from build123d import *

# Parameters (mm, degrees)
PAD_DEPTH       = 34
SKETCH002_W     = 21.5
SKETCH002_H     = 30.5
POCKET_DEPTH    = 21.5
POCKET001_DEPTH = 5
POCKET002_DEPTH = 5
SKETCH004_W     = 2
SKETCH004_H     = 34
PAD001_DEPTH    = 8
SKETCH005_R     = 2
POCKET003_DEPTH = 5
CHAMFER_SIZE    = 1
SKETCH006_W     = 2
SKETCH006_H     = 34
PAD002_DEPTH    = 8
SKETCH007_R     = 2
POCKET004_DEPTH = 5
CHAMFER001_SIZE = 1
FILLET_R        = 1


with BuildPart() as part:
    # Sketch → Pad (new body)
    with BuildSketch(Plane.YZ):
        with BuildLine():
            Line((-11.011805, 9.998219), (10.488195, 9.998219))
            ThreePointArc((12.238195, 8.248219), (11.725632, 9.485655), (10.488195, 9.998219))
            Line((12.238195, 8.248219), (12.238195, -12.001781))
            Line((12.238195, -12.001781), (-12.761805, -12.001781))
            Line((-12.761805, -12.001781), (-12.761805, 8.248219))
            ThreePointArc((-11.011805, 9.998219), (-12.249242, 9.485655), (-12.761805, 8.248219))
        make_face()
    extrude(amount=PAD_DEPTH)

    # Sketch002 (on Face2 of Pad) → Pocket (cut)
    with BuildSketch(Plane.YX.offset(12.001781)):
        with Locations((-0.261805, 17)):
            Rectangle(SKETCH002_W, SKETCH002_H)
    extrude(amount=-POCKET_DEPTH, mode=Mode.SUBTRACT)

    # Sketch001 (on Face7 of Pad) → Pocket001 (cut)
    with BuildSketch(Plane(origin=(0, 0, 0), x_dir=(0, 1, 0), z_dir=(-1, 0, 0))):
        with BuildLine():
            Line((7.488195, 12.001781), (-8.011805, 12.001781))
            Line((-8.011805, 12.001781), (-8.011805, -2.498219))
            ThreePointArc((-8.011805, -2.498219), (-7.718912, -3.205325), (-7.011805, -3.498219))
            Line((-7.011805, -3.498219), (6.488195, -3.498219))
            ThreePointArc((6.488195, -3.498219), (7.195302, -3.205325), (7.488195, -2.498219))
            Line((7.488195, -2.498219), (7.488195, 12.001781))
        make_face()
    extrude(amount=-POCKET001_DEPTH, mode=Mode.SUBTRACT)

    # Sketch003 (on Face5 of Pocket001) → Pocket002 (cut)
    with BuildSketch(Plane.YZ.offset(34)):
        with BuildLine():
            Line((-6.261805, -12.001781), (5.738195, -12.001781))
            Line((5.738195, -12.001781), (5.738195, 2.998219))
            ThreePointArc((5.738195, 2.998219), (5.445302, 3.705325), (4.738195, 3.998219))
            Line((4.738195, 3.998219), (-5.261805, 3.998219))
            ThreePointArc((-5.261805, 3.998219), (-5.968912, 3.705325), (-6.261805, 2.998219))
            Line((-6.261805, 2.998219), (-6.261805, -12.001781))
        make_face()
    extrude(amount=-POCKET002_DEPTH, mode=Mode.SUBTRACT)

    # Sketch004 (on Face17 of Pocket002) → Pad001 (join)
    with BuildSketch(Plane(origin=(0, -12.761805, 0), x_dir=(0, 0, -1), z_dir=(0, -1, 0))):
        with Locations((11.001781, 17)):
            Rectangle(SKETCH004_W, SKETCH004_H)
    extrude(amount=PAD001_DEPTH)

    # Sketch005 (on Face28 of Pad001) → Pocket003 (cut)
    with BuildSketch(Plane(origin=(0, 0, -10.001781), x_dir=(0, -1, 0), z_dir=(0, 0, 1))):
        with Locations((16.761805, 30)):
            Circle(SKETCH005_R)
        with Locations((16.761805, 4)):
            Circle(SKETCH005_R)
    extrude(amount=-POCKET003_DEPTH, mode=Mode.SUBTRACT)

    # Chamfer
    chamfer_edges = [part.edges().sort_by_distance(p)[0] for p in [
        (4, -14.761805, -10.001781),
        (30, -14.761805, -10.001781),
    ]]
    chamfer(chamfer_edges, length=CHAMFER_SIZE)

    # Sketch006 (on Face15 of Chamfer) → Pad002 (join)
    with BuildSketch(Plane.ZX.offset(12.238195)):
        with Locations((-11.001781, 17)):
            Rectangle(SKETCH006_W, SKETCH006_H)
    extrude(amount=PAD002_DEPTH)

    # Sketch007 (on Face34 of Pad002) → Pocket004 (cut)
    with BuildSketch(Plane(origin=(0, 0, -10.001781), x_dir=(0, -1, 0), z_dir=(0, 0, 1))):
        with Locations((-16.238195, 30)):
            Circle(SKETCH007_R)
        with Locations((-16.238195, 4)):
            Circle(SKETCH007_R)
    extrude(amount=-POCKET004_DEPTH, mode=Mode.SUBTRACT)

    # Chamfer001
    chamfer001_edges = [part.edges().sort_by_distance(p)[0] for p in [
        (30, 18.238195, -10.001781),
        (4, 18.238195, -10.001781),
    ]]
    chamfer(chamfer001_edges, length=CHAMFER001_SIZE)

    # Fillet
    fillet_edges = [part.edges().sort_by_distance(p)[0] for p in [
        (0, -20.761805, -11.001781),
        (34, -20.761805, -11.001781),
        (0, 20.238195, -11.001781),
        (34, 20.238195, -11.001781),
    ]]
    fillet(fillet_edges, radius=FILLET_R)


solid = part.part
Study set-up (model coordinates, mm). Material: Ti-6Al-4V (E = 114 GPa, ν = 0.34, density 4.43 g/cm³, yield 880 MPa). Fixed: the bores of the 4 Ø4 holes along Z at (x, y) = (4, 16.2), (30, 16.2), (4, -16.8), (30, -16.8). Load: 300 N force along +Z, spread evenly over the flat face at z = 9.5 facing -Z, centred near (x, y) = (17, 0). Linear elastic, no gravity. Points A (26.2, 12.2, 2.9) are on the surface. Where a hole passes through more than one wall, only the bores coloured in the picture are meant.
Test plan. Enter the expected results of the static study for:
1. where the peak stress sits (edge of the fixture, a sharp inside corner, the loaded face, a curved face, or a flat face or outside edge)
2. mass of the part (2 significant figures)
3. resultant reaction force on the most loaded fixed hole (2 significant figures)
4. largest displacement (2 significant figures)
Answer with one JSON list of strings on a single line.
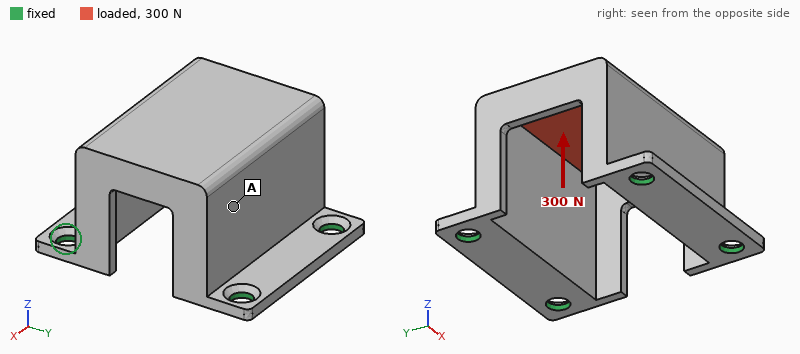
["a curved face", "21 g", "80 N", "0.17 mm"]
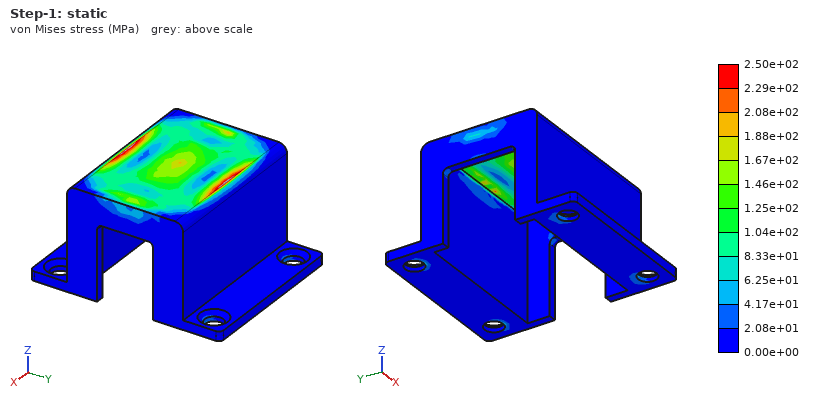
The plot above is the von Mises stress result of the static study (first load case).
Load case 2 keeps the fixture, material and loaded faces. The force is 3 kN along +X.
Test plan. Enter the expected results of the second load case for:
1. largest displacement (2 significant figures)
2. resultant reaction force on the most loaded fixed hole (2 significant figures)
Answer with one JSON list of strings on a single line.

["86 µm", "1.5 kN"]
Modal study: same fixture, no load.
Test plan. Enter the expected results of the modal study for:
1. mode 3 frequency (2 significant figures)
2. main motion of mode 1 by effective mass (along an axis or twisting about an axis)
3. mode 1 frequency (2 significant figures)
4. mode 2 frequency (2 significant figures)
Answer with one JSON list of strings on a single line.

["9900 Hz", "along Y", "6400 Hz", "7000 Hz"]
